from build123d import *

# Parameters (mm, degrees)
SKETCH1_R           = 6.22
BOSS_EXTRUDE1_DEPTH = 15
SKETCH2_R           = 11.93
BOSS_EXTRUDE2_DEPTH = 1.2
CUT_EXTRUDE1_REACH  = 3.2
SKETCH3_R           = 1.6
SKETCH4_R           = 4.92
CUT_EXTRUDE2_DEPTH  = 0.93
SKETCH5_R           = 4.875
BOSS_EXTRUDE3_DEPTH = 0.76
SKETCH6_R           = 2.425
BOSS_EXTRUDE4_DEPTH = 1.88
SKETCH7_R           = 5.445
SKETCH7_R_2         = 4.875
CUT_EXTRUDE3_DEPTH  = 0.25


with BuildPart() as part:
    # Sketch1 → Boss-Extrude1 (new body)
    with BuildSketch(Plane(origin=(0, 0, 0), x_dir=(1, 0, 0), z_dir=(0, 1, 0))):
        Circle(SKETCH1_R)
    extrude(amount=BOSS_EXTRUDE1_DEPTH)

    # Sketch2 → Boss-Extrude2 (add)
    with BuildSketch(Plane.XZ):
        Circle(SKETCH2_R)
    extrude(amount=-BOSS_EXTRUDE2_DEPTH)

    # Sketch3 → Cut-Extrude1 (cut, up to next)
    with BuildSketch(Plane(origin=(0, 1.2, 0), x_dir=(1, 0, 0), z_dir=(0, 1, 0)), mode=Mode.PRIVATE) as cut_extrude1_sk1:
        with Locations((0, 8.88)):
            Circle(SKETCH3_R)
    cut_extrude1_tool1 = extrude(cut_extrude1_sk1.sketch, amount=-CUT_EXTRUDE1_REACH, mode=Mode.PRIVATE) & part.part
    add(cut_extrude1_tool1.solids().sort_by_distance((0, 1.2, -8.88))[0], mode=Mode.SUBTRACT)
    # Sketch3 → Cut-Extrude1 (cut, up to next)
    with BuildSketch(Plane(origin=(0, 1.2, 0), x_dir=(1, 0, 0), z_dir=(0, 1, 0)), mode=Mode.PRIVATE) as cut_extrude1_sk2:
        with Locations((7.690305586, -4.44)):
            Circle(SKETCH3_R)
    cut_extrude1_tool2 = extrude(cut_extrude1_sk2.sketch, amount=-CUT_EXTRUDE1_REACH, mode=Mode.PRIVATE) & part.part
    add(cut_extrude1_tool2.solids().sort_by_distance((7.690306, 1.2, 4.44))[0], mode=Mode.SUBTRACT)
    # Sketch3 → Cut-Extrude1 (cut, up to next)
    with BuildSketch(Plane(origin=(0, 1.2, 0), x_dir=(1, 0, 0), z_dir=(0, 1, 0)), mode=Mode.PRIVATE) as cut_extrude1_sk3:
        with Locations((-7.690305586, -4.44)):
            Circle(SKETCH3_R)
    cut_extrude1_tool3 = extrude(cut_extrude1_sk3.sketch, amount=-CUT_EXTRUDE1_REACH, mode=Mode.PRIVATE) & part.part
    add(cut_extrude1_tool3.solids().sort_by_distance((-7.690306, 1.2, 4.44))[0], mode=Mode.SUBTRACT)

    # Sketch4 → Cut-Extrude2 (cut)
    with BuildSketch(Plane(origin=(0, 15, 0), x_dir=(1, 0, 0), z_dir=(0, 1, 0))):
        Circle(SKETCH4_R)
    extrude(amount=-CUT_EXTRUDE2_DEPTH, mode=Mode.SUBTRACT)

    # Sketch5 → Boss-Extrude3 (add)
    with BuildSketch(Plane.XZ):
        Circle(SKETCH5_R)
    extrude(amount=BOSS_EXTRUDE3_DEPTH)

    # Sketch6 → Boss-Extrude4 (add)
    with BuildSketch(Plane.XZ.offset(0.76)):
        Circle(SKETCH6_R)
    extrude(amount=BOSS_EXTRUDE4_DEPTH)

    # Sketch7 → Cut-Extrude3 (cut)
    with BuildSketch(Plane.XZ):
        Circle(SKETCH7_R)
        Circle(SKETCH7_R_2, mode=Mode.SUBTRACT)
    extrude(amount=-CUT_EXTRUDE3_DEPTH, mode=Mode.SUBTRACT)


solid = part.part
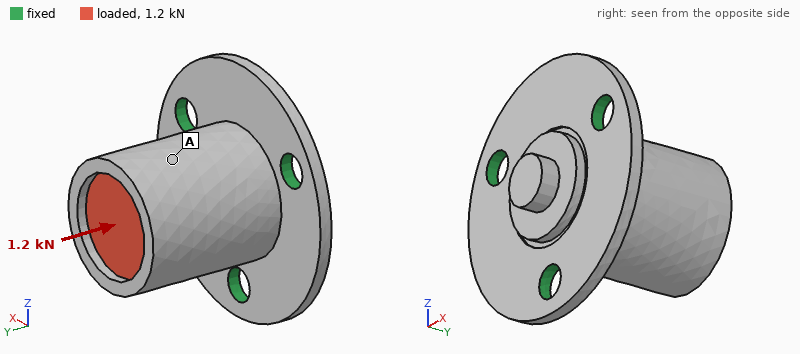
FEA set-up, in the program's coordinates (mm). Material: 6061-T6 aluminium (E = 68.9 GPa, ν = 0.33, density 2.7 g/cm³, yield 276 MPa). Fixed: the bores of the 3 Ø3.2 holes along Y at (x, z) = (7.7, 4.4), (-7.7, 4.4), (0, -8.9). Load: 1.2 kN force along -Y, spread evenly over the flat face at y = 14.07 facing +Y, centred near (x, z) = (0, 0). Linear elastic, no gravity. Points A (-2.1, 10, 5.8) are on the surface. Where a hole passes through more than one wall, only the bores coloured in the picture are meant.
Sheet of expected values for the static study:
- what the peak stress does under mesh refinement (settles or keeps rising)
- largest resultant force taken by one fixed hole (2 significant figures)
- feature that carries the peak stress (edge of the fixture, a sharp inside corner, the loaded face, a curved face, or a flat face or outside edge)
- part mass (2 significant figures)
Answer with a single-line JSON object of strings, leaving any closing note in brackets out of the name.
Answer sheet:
{"what the peak stress does under mesh refinement": "keeps rising", "largest resultant force taken by one fixed hole": "440 N", "feature that carries the peak stress": "edge of the fixture", "part mass": "5.9 g"}
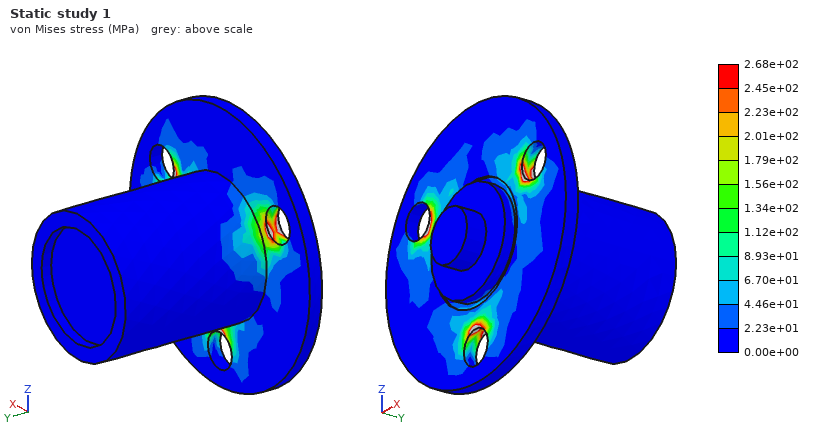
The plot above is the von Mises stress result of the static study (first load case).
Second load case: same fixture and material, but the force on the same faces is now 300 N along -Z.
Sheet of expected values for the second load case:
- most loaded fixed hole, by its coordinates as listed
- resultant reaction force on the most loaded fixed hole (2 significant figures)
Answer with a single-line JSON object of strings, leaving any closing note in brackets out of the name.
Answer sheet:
{"most loaded fixed hole, by its coordinates as listed": "(0, -8.9)", "resultant reaction force on the most loaded fixed hole": "410 N"}
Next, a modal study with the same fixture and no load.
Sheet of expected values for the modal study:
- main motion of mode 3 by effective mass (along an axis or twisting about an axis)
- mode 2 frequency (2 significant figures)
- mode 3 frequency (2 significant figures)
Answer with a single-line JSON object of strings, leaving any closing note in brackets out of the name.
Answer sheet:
{"main motion of mode 3 by effective mass": "along Y", "mode 2 frequency": "13 kHz", "mode 3 frequency": "22 kHz"}
